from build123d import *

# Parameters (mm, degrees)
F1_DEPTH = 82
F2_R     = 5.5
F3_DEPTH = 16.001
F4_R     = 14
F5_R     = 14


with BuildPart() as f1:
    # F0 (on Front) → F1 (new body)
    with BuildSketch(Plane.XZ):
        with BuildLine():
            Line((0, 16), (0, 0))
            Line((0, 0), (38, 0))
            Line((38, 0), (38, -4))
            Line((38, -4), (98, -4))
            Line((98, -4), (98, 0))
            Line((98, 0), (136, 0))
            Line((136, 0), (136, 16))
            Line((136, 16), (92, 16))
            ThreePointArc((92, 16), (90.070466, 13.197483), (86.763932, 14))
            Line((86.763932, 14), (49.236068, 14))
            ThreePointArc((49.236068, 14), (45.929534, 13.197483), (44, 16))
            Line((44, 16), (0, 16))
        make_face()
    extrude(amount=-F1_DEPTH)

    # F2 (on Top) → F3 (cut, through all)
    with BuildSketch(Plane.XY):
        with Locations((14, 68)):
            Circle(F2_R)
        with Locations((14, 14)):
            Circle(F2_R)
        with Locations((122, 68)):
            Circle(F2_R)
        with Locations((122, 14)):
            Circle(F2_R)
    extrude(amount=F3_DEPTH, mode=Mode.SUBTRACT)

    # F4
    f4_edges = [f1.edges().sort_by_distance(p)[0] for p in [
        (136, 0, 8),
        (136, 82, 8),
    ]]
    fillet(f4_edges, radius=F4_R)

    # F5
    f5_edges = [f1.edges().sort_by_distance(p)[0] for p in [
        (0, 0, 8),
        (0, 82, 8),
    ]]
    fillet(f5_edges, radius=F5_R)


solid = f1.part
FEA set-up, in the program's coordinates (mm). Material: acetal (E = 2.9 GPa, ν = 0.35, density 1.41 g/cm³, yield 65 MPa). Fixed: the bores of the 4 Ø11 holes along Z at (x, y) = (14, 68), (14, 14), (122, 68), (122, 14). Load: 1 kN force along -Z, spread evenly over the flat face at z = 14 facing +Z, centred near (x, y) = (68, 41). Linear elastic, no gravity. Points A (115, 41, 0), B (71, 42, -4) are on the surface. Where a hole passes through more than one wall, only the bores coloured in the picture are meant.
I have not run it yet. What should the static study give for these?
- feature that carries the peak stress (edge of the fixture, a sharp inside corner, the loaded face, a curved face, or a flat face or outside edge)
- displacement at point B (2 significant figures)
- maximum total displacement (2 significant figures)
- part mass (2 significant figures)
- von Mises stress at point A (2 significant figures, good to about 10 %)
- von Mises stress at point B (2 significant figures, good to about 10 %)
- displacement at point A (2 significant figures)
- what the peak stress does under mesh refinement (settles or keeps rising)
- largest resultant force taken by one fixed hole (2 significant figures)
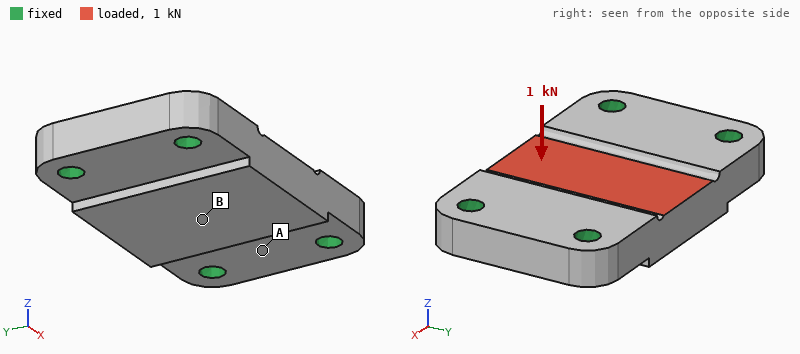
edge of the fixture
68 µm
77 µm
260 g
0.74 MPa
2.1 MPa
14 µm
keeps rising
290 N
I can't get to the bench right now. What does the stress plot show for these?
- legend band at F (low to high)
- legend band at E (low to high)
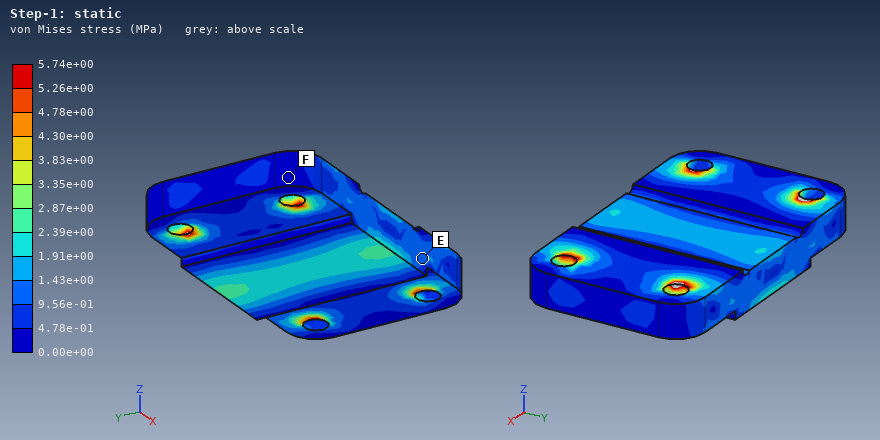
0.00e+00 to 4.78e-01 MPa
9.56e-01 to 1.43e+00 MPa
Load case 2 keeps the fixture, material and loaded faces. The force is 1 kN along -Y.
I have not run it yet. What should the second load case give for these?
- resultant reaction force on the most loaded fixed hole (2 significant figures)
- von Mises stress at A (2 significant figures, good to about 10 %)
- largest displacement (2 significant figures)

300 N
0.42 MPa
38 µm
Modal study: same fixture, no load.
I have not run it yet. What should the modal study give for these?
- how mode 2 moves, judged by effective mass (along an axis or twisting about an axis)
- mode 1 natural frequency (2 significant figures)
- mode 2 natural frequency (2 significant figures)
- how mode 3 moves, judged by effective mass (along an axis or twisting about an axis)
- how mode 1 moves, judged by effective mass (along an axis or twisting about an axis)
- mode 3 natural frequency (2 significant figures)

twisting about X
1800 Hz
2400 Hz
along Y
along Z
3400 Hz
